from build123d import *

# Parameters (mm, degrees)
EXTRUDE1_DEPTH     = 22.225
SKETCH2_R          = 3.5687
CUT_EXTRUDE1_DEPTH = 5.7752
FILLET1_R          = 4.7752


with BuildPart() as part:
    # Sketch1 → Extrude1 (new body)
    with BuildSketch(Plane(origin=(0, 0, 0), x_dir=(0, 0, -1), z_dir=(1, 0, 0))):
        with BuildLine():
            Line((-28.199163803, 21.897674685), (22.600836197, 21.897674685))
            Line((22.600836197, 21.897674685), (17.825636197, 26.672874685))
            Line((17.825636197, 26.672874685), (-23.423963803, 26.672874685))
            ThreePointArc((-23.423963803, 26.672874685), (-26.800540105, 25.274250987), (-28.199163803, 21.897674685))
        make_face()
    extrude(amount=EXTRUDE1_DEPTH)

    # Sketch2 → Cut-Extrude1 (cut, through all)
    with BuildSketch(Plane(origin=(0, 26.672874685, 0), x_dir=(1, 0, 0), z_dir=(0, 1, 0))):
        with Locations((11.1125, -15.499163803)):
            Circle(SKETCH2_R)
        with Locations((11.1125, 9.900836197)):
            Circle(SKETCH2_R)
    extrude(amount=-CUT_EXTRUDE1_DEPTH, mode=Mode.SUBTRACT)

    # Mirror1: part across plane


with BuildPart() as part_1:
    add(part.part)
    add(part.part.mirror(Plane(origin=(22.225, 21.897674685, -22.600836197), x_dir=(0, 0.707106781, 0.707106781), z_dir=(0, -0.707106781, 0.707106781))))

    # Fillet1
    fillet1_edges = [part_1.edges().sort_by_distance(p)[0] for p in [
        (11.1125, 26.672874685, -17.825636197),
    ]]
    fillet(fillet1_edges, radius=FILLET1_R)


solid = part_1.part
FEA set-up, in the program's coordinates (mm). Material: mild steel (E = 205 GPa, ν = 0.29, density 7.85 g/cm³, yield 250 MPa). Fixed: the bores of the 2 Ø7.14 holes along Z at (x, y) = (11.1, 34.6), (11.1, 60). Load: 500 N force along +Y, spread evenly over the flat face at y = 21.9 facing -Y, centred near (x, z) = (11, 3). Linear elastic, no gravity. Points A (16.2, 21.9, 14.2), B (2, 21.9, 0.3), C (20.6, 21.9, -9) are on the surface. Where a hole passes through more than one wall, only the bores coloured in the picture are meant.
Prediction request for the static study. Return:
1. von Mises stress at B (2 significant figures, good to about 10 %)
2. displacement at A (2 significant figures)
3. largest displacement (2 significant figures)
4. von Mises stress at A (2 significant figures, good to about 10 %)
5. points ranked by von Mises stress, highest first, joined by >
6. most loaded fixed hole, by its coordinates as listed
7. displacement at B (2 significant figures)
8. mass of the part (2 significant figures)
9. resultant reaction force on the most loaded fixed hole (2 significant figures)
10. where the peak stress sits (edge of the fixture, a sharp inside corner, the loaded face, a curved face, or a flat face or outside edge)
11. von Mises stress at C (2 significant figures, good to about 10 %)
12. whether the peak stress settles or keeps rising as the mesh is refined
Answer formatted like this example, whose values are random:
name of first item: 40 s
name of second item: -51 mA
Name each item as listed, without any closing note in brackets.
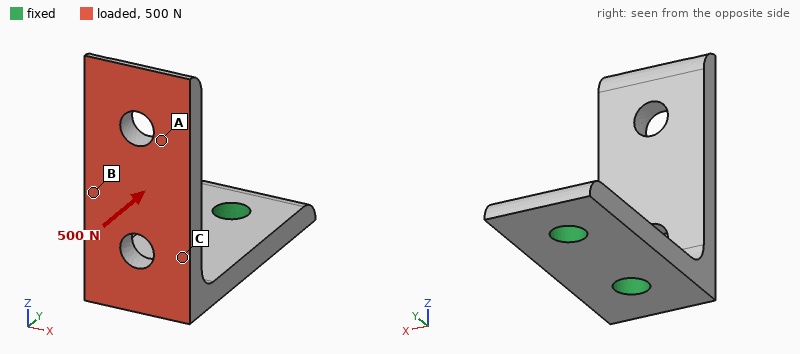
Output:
von Mises stress at B: 49 MPa
displacement at A: 0.14 mm
largest displacement: 0.23 mm
von Mises stress at A: 18 MPa
points ranked by von Mises stress, highest first, joined by >: C > B > A
most loaded fixed hole, by its coordinates as listed: (11.1, 34.6)
displacement at B: 0.069 mm
mass of the part: 74 g
resultant reaction force on the most loaded fixed hole: 480 N
where the peak stress sits: edge of the fixture
von Mises stress at C: 110 MPa
whether the peak stress settles or keeps rising as the mesh is refined: keeps rising
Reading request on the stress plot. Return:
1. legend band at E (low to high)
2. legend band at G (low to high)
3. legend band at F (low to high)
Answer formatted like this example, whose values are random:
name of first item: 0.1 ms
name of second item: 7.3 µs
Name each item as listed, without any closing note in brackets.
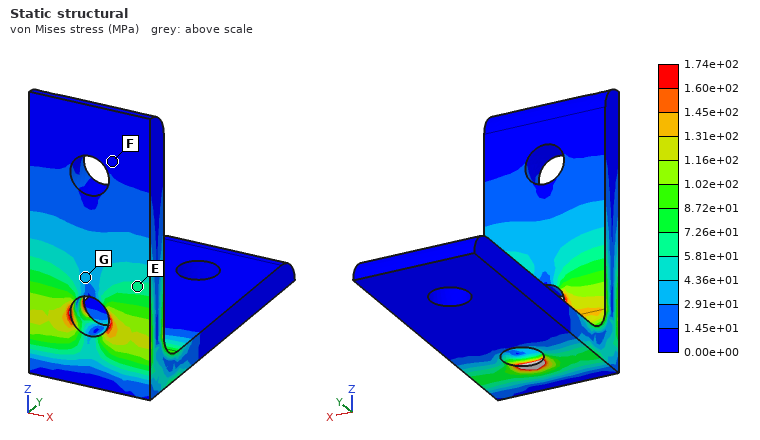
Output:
legend band at E: 5.81e+01 to 7.26e+01 MPa
legend band at G: 2.91e+01 to 4.36e+01 MPa
legend band at F: 0.00e+00 to 1.45e+01 MPa
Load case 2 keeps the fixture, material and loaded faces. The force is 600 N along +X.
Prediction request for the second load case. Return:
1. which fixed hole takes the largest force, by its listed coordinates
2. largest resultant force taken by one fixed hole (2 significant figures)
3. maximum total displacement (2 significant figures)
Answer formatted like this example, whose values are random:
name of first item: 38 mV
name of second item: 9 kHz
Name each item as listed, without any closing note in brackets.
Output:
which fixed hole takes the largest force, by its listed coordinates: (11.1, 34.6)
largest resultant force taken by one fixed hole: 720 N
maximum total displacement: 61 µm
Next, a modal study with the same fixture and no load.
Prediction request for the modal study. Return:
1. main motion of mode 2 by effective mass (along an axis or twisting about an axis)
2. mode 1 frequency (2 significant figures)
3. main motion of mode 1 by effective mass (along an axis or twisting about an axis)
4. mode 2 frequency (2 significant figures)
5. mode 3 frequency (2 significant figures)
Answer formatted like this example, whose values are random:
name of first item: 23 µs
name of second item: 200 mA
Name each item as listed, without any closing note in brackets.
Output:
main motion of mode 2 by effective mass: along X
mode 1 frequency: 1500 Hz
main motion of mode 1 by effective mass: along Y
mode 2 frequency: 3100 Hz
mode 3 frequency: 7000 Hz
